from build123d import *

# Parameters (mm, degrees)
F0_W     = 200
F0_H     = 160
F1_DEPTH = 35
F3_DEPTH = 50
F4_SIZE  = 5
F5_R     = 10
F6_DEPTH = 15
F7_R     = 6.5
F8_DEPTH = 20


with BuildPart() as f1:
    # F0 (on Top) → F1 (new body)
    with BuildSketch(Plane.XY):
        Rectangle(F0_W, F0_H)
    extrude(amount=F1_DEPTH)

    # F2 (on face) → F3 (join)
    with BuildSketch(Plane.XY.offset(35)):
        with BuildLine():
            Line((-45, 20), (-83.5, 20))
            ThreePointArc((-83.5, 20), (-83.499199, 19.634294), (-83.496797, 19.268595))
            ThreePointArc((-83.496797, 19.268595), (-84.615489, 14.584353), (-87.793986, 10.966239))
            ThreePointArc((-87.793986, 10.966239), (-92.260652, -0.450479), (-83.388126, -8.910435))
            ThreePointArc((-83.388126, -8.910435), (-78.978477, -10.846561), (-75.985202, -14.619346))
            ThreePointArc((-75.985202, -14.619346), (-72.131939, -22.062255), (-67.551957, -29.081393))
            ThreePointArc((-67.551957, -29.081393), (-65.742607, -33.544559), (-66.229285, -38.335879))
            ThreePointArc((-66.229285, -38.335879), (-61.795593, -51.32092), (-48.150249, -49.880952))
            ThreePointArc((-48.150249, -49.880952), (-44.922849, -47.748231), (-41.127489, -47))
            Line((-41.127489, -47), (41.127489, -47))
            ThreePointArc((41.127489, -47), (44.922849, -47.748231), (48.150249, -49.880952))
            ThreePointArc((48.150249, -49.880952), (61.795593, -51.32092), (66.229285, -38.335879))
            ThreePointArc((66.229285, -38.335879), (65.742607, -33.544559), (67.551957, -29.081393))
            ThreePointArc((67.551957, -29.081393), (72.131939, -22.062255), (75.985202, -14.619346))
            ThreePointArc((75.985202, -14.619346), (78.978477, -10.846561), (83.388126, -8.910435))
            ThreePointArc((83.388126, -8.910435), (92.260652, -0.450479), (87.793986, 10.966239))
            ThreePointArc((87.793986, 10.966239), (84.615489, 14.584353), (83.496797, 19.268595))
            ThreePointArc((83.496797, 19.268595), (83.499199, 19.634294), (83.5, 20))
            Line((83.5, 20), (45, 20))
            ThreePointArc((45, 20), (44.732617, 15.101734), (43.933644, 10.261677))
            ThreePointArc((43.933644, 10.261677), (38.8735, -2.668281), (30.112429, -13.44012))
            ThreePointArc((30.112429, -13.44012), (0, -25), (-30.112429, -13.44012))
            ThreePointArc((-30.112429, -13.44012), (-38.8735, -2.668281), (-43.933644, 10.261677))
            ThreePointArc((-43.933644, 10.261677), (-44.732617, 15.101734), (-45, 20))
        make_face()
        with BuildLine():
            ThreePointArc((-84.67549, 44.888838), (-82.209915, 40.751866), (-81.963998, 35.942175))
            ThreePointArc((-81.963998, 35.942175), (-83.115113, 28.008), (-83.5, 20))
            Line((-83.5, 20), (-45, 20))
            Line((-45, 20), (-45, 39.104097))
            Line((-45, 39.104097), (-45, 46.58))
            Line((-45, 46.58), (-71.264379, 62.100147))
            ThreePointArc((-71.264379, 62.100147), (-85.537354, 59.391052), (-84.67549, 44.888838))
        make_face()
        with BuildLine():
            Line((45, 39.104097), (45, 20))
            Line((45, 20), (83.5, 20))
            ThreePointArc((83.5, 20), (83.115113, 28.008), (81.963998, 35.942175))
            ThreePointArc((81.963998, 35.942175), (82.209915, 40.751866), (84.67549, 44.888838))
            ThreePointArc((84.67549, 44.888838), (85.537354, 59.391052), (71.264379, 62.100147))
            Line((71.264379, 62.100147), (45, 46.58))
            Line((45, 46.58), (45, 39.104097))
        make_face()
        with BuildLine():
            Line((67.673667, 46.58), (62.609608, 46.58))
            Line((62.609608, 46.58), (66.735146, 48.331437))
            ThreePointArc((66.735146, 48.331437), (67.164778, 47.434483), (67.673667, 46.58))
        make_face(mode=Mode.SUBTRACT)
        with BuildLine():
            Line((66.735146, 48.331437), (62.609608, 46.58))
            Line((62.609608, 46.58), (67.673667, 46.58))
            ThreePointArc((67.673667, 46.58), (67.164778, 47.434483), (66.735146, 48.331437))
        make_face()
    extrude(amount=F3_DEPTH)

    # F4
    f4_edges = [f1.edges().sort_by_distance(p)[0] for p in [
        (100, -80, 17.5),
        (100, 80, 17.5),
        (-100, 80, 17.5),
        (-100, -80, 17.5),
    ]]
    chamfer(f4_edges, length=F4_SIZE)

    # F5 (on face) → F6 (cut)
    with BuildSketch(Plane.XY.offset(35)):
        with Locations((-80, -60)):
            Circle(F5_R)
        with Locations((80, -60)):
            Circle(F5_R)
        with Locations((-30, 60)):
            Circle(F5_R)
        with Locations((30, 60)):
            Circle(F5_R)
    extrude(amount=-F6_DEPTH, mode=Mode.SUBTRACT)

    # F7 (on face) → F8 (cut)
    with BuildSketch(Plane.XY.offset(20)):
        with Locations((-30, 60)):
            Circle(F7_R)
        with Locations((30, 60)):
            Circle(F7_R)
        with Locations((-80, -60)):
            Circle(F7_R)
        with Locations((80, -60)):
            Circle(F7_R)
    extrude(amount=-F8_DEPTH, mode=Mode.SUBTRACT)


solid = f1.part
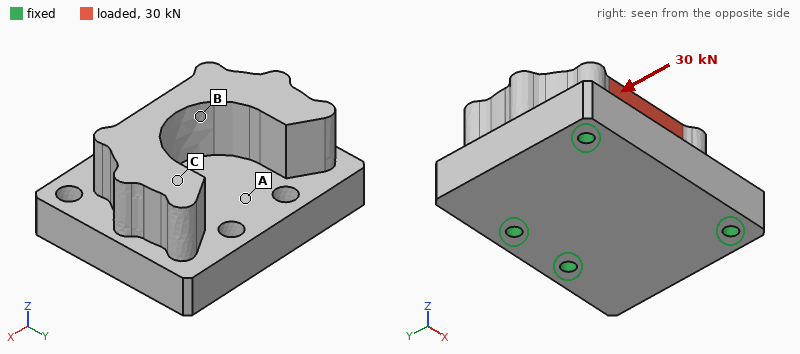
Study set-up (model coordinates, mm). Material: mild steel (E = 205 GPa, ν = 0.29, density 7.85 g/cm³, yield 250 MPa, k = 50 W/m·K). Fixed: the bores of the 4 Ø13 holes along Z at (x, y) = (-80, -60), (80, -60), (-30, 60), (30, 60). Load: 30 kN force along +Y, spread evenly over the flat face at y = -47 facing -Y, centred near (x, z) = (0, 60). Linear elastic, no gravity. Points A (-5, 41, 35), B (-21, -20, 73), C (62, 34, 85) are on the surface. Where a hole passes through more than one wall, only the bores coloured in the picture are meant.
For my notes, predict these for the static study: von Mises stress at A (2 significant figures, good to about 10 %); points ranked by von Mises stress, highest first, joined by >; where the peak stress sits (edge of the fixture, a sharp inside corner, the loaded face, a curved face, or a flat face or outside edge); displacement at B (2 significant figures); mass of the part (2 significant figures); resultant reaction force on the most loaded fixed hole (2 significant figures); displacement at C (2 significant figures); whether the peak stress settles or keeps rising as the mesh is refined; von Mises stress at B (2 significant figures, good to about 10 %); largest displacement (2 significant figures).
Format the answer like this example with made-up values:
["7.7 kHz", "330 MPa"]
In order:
["7.3 MPa", "B > A > C", "edge of the fixture", "11 µm", "13 kg", "11 kN", "8.7 µm", "keeps rising", "13 MPa", "18 µm"]
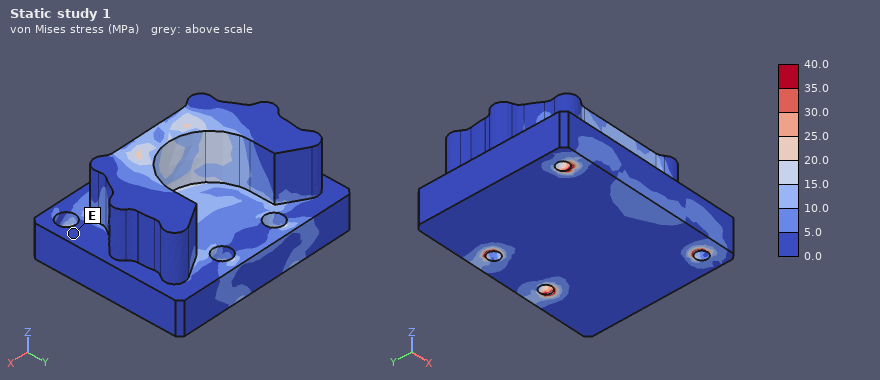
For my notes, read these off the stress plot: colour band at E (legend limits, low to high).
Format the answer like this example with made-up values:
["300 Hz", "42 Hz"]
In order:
["0.0 to 5.0 MPa"]
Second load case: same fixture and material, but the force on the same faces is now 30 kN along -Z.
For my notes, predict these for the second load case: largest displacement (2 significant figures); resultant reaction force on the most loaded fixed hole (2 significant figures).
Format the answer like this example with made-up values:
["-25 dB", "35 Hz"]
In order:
["18 µm", "15 kN"]
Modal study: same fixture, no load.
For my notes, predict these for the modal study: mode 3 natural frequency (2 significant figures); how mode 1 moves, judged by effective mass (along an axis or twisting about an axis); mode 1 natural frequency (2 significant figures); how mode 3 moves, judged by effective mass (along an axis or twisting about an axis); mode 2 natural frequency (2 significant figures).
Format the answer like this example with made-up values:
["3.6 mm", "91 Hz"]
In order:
["4300 Hz", "along X", "3500 Hz", "along Z", "3800 Hz"]
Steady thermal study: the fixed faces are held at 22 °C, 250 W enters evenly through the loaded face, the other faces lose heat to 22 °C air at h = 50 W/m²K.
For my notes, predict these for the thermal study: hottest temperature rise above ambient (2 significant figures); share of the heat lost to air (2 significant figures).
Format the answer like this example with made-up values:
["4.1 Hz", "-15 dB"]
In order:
["72 K", "38 %"]
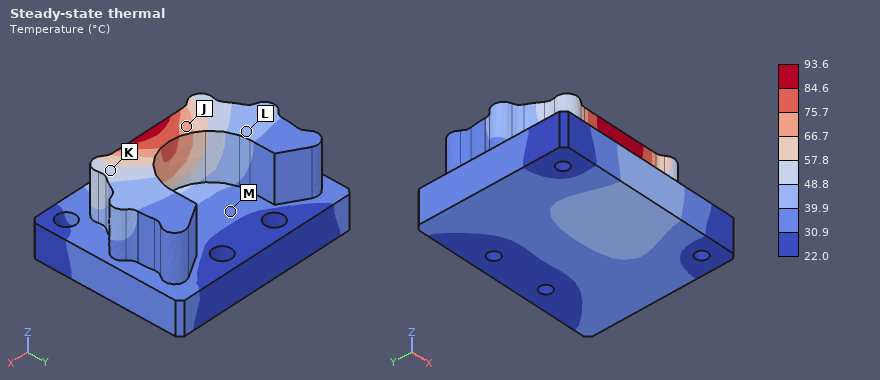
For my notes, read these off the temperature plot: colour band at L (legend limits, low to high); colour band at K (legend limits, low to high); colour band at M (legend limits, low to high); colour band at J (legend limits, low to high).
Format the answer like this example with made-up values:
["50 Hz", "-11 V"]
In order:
["39.9 to 48.8 °C", "48.8 to 57.8 °C", "30.9 to 39.9 °C", "66.7 to 75.7 °C"]
